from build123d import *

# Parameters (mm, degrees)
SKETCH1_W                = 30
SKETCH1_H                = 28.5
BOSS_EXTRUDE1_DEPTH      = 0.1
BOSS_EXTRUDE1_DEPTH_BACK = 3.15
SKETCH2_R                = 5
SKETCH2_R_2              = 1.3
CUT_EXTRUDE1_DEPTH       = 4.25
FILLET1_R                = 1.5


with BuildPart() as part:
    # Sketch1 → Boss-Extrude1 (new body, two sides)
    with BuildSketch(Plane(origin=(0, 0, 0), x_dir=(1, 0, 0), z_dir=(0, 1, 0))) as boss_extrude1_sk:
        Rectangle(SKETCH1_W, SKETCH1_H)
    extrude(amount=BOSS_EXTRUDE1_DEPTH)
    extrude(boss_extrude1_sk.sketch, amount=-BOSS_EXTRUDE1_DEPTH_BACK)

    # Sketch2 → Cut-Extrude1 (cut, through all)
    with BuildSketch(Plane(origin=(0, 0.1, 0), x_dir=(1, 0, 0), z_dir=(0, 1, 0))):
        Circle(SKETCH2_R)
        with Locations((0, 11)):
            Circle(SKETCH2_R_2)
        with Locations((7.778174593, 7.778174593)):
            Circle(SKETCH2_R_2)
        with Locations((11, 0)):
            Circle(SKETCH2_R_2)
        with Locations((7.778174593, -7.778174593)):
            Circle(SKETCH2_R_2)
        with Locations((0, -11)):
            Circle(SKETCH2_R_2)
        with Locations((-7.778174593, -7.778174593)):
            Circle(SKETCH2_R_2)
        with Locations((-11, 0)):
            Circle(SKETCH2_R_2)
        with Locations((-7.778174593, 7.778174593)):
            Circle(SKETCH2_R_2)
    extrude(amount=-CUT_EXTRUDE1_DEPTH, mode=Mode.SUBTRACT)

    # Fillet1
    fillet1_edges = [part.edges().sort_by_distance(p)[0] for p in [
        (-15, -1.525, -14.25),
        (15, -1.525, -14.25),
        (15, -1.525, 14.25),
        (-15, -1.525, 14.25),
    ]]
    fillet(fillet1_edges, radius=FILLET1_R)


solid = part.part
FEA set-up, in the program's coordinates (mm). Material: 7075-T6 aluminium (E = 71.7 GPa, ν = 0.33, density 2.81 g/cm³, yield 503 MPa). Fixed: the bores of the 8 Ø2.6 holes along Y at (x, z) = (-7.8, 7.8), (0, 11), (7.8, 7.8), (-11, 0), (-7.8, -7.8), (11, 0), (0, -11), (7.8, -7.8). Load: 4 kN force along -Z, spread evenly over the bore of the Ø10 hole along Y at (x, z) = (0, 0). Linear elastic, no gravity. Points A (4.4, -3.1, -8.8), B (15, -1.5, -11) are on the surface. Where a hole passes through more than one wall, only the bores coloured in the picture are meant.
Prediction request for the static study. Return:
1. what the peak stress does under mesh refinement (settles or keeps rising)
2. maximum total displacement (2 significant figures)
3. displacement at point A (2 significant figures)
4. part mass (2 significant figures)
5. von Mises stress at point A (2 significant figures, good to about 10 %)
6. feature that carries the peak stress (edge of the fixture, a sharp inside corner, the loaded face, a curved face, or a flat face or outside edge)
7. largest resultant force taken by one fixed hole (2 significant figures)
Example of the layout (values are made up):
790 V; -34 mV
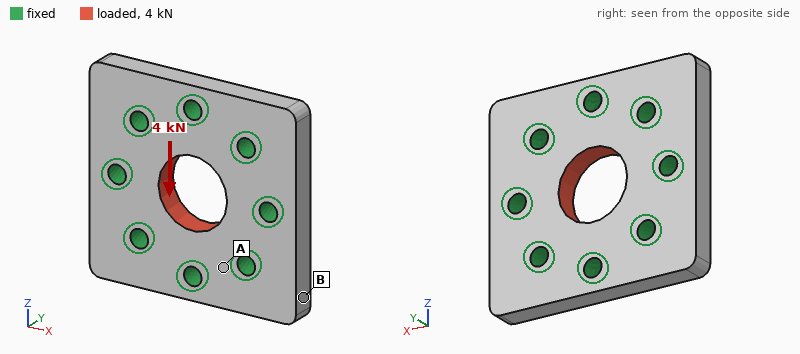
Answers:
keeps rising; 3.5 µm; 1.2 µm; 6.7 g; 15 MPa; edge of the fixture; 790 N
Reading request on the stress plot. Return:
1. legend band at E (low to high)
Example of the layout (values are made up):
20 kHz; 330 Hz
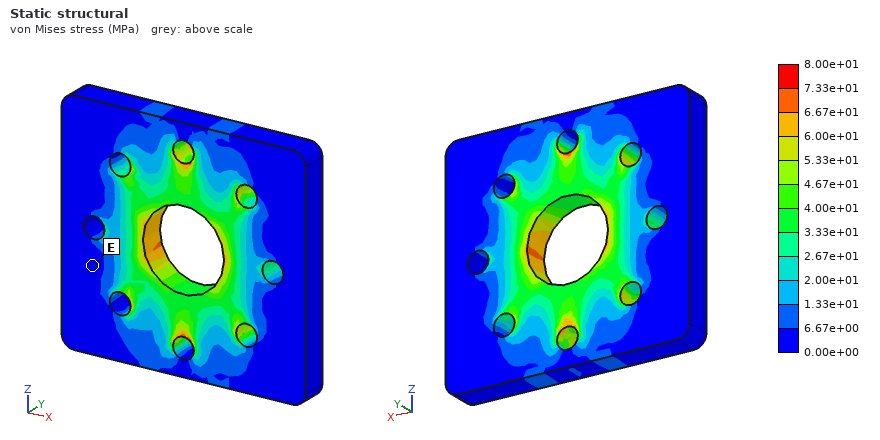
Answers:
0.00e+00 to 6.67e+00 MPa
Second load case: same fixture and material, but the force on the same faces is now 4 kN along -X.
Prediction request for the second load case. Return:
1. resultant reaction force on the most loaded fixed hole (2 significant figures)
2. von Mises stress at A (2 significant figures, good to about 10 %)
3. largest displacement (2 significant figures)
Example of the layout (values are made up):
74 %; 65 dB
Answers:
790 N; 10 MPa; 3.5 µm
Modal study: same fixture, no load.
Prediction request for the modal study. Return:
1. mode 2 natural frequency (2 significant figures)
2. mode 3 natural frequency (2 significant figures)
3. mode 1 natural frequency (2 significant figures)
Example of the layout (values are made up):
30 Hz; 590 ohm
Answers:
46 kHz; 46 kHz; 46 kHz
